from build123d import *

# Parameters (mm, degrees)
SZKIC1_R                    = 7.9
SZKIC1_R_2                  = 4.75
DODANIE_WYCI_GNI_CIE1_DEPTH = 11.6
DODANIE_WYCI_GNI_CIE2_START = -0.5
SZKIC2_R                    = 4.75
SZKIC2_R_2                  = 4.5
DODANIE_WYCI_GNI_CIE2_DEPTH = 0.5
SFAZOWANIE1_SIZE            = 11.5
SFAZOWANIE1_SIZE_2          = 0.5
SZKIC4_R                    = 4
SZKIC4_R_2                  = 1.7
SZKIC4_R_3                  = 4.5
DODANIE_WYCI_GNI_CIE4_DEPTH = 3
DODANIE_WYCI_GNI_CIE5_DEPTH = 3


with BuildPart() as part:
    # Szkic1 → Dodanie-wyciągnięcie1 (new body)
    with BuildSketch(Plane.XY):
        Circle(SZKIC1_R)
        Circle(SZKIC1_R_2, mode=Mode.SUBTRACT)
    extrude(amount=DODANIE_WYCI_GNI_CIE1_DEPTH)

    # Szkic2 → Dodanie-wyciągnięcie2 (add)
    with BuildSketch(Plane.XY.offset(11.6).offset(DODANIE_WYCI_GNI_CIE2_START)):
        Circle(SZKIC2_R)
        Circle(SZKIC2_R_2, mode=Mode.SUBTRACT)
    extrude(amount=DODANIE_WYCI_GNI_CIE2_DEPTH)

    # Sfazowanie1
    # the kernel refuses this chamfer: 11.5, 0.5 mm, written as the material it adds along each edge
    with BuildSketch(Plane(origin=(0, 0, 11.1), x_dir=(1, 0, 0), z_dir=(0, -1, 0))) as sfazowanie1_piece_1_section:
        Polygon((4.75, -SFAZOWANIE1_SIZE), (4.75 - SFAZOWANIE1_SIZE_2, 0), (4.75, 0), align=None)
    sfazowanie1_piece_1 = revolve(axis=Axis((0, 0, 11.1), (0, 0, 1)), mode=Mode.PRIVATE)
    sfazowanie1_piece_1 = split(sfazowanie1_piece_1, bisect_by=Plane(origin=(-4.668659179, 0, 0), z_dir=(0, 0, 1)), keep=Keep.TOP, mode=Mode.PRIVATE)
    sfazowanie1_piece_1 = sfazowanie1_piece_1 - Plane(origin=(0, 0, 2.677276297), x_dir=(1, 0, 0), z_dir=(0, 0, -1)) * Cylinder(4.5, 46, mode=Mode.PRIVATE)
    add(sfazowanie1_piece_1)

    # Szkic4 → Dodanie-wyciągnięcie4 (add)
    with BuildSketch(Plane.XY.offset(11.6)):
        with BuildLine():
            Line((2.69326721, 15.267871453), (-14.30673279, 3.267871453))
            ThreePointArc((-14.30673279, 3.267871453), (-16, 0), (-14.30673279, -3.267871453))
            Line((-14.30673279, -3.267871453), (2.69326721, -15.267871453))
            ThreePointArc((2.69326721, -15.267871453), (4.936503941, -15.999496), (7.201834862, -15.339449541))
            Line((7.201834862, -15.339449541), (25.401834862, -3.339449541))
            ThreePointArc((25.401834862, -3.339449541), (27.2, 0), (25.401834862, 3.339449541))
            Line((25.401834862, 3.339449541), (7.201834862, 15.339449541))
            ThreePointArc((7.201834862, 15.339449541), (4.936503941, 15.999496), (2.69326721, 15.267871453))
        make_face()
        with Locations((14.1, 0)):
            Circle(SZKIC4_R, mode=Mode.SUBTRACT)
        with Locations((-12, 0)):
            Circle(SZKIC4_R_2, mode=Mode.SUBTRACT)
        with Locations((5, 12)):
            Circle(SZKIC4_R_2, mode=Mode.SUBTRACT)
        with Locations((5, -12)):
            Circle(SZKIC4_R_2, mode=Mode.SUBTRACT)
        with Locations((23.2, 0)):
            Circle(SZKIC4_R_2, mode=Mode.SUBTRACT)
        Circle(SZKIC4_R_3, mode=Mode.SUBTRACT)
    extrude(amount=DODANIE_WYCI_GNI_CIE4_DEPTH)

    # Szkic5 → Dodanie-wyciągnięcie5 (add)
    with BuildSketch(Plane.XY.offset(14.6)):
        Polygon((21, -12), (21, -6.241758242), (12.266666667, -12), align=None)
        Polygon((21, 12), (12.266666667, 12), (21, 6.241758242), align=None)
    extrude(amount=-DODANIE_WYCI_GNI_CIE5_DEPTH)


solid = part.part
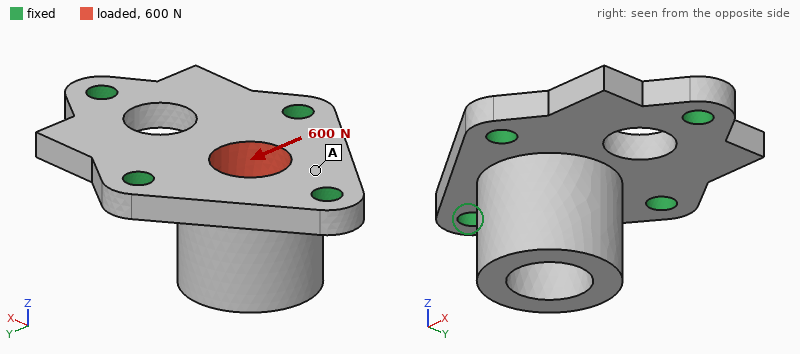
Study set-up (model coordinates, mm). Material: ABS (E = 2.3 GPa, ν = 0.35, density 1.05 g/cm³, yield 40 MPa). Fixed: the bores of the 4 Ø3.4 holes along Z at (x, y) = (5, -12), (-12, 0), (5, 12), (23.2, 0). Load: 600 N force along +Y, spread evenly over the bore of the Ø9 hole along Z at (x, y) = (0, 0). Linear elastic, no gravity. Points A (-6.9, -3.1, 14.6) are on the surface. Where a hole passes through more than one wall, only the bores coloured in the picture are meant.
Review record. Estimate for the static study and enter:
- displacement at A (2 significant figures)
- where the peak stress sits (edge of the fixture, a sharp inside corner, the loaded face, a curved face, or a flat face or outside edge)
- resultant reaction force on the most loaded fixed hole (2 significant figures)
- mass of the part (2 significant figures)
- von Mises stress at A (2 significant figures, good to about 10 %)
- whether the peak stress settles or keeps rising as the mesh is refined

0.031 mm
edge of the fixture
240 N
3.8 g
2.7 MPa
keeps rising
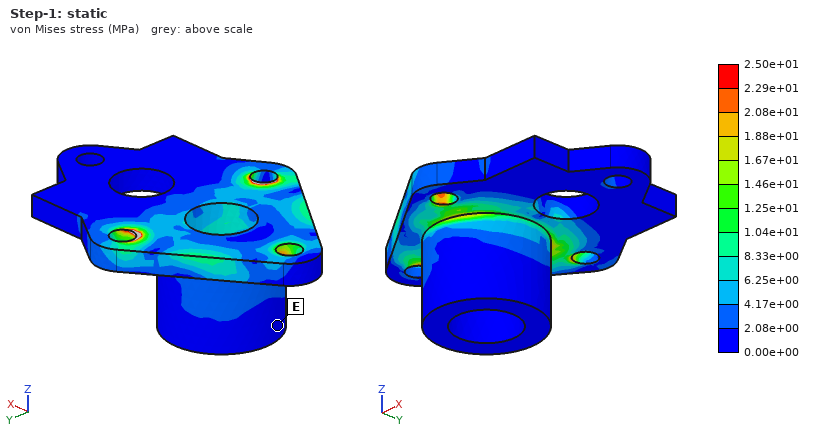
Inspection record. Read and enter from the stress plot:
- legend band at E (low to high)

0.00e+00 to 2.08e+00 MPa
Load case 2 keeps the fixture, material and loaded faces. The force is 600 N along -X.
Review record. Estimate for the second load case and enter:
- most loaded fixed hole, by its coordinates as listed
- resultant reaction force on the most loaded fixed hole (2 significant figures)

(-12, 0)
270 N
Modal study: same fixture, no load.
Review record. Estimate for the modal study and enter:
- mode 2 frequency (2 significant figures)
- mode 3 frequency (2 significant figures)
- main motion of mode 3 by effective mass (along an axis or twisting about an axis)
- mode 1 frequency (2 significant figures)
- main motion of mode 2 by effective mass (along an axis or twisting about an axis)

6200 Hz
7700 Hz
along Z
5800 Hz
along Y
